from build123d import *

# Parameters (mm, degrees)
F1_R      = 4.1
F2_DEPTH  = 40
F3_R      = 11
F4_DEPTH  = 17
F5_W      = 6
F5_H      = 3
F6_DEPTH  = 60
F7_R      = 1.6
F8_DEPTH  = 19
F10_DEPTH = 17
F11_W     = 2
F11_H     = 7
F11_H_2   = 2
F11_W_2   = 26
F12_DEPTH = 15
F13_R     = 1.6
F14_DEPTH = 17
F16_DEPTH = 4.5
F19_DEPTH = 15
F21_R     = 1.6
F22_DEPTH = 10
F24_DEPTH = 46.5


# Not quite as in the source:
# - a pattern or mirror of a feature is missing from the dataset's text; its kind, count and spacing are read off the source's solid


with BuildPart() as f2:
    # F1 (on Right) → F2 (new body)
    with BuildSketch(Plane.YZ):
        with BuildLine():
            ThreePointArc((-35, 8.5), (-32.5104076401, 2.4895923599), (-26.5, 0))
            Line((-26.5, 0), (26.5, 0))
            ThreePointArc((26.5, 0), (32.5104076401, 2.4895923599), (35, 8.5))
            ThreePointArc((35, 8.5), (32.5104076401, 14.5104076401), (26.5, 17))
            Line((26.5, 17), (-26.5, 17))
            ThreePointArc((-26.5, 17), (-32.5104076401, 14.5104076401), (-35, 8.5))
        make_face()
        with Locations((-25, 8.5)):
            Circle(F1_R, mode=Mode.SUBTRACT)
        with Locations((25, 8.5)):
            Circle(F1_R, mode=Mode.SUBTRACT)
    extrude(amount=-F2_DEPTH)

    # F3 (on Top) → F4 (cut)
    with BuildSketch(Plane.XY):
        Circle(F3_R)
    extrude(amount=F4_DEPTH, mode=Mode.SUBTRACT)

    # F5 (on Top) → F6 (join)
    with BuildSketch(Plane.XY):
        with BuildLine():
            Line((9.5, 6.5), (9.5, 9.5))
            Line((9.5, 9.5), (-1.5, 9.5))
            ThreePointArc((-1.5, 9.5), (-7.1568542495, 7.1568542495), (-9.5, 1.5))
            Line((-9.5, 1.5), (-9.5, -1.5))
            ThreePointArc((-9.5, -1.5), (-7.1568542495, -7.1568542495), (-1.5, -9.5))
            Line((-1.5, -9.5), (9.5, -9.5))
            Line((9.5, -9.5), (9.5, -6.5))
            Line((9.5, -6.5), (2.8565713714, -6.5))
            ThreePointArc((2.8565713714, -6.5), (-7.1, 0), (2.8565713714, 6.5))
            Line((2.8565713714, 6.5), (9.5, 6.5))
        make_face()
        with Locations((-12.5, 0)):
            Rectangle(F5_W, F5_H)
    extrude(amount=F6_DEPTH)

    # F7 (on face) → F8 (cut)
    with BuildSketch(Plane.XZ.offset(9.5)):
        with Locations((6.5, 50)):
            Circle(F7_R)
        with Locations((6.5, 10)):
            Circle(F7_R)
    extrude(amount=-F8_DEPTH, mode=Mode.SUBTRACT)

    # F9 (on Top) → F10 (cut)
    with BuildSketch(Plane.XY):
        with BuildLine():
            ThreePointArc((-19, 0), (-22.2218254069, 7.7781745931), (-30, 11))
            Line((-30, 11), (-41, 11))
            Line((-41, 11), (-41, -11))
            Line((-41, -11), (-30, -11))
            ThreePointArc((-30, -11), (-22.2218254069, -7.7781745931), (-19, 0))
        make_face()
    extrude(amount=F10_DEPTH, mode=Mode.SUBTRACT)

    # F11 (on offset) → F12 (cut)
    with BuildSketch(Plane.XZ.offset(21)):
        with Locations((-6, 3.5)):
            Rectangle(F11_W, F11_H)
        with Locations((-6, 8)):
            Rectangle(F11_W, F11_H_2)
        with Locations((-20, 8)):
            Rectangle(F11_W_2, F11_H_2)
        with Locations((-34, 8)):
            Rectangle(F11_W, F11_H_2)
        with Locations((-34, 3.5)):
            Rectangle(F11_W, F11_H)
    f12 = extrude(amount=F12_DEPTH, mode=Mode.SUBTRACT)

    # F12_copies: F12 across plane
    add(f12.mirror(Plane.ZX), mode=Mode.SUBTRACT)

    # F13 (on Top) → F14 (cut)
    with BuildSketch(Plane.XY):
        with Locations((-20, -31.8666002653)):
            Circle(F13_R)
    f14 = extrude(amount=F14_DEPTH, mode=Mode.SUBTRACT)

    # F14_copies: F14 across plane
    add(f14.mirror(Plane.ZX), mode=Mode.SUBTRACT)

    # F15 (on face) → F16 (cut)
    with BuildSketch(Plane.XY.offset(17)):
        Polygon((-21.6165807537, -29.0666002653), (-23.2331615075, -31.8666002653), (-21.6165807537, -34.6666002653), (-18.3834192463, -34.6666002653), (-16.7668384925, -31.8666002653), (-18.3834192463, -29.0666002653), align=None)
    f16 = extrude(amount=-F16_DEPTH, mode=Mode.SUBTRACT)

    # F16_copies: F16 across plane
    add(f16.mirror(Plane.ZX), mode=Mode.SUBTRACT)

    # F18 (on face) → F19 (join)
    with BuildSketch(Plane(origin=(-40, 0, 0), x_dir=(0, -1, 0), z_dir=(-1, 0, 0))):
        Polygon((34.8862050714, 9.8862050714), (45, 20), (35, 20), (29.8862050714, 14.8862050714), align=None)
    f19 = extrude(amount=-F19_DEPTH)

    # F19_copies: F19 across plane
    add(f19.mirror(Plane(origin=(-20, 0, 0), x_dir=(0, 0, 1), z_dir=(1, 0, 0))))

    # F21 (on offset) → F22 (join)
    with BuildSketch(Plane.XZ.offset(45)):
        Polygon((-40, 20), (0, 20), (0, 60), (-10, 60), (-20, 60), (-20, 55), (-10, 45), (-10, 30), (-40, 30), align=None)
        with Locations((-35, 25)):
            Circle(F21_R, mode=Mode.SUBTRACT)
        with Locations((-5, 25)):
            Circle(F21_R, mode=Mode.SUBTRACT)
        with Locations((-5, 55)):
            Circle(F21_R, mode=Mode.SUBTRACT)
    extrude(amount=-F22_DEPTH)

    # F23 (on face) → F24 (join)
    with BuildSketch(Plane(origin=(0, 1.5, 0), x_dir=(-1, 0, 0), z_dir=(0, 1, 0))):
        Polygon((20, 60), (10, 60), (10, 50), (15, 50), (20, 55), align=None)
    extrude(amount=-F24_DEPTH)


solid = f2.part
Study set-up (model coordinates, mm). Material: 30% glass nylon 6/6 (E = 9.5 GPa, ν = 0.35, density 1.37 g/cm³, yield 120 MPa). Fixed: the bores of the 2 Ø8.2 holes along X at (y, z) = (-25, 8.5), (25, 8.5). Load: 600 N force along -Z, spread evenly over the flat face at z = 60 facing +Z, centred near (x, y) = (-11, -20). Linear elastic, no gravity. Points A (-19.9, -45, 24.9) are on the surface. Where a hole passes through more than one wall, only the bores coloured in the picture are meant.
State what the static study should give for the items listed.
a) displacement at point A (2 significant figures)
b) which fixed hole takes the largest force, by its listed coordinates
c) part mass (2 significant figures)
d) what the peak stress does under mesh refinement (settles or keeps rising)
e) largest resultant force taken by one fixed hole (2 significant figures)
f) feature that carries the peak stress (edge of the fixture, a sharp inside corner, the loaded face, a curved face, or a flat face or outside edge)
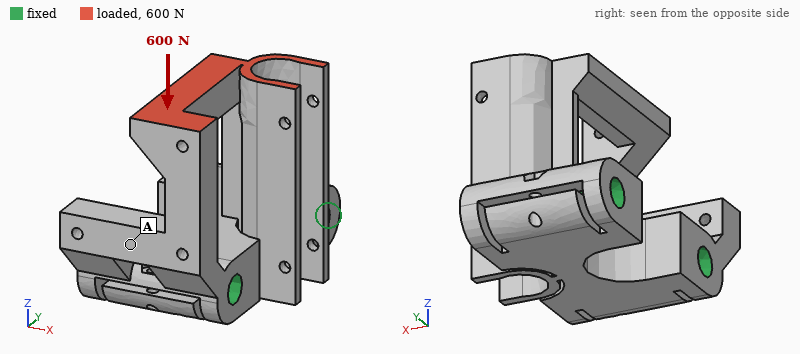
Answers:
0.034 mm
(-25, 8.5)
69 g
keeps rising
470 N
a sharp inside corner
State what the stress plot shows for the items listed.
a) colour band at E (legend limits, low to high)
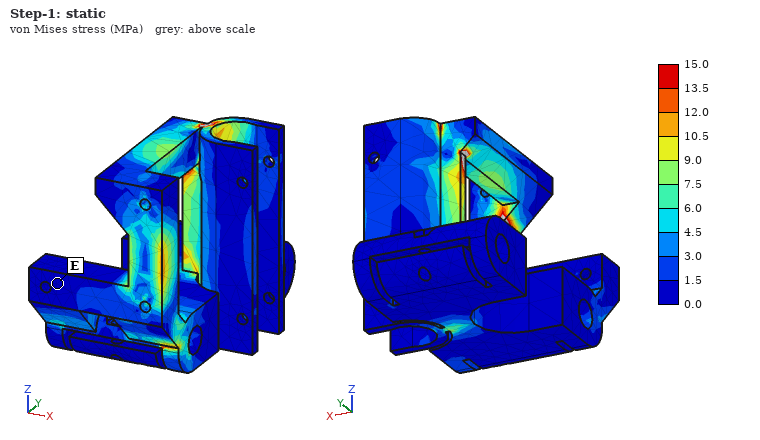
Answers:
0.0 to 1.5 MPa
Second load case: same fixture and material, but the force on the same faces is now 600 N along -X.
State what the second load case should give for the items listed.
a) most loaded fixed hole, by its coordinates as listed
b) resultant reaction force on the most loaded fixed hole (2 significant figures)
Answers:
(-25, 8.5)
470 N
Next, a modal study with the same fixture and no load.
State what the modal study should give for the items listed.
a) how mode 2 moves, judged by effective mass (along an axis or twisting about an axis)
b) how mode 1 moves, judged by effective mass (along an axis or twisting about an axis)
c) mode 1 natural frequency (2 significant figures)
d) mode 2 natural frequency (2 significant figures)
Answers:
along X
along Y
1200 Hz
1300 Hz
